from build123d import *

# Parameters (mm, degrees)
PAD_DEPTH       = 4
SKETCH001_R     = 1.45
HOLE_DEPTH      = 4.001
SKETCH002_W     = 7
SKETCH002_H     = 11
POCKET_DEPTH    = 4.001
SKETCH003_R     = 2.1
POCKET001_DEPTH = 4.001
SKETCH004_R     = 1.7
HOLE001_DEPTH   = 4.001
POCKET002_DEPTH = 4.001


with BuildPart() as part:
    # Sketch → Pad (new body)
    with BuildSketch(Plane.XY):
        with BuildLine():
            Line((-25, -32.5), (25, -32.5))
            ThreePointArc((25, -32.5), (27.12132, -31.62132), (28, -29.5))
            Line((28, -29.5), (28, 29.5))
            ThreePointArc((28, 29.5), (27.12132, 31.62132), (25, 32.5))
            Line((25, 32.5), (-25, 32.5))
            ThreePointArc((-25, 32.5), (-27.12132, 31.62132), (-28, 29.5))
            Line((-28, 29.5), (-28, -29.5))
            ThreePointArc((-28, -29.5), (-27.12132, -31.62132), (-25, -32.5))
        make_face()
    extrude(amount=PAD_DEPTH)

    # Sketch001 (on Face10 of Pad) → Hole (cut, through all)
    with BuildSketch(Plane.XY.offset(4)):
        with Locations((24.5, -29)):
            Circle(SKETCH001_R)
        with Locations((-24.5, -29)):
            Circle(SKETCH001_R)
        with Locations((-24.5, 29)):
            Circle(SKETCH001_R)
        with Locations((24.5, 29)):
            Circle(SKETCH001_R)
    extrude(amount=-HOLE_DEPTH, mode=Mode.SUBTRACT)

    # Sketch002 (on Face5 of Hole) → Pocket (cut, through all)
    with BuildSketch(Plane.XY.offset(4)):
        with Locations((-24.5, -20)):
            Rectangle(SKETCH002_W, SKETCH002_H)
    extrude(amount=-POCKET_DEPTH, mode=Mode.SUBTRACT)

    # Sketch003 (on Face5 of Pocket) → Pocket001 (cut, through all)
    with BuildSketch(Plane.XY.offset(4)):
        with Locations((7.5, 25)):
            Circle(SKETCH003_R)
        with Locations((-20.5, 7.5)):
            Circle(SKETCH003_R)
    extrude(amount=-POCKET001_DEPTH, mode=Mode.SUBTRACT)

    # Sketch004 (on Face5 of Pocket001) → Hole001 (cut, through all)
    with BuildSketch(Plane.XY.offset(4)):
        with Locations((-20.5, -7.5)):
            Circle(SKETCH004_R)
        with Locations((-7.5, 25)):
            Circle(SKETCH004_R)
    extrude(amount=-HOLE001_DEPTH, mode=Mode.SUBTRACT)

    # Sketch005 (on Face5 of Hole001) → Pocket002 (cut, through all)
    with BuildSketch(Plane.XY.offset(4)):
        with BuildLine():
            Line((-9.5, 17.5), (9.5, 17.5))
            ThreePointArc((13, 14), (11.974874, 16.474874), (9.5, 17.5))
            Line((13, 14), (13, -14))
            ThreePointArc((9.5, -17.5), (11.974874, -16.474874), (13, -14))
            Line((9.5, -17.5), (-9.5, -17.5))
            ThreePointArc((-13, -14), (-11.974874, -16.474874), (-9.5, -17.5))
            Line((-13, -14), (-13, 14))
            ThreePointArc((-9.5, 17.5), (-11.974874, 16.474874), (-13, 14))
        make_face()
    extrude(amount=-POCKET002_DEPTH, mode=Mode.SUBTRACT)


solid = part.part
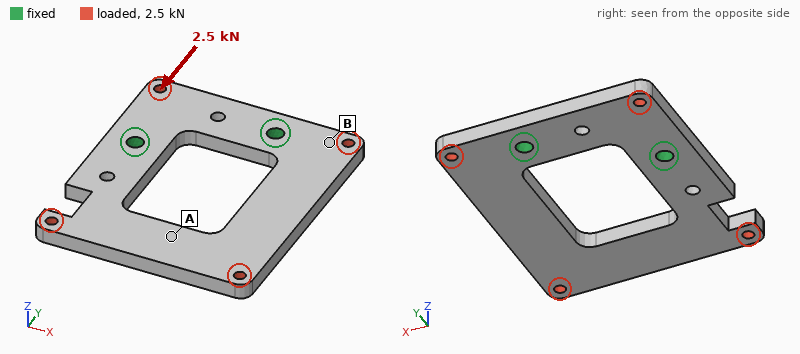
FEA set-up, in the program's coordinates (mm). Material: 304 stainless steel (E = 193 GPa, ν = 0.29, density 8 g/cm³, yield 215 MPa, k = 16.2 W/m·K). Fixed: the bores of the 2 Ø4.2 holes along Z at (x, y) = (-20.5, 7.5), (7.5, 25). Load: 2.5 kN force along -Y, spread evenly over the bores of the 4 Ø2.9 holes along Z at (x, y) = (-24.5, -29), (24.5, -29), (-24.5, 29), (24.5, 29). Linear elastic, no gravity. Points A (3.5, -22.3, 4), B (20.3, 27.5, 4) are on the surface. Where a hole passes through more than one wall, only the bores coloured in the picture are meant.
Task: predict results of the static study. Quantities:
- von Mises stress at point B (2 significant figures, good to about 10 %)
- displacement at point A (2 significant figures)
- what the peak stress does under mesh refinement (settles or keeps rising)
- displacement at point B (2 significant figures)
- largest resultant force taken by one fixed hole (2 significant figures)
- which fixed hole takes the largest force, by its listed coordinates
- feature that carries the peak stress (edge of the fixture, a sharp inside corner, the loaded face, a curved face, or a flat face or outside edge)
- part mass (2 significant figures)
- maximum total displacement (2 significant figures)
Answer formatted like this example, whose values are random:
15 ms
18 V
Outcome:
19 MPa
13 µm
keeps rising
8.1 µm
1.4 kN
(7.5, 25)
edge of the fixture
83 g
19 µm
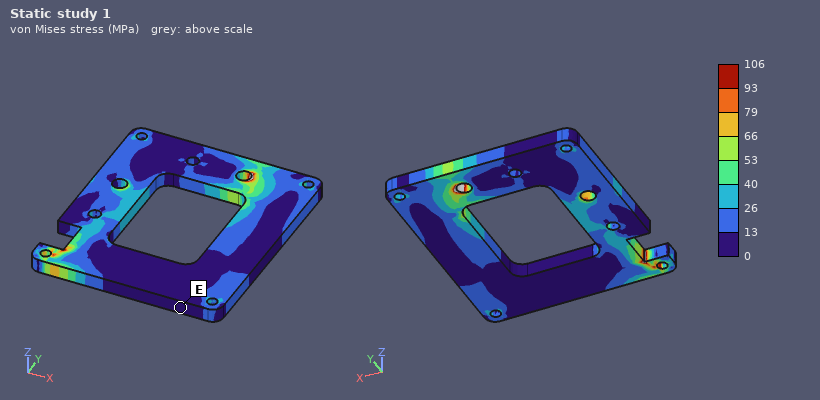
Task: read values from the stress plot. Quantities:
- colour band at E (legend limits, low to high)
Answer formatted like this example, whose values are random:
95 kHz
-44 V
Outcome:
0 to 13 MPa
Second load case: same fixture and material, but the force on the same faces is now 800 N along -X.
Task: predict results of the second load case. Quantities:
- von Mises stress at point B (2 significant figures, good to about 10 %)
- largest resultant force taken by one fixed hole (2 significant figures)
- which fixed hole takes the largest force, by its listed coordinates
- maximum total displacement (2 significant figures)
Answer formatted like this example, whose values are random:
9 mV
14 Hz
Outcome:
9.0 MPa
530 N
(-20.5, 7.5)
14 µm
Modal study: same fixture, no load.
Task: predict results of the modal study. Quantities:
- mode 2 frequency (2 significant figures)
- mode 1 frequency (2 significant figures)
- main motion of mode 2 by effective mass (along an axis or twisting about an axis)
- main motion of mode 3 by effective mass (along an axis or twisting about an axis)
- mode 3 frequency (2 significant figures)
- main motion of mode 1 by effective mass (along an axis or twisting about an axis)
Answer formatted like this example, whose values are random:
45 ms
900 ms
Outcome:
2500 Hz
980 Hz
twisting about Y
along X
4800 Hz
along Z
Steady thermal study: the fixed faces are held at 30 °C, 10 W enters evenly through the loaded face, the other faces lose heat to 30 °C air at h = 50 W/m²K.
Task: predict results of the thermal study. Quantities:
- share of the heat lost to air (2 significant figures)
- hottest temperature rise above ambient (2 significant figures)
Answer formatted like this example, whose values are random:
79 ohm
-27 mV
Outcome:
64 %
74 K
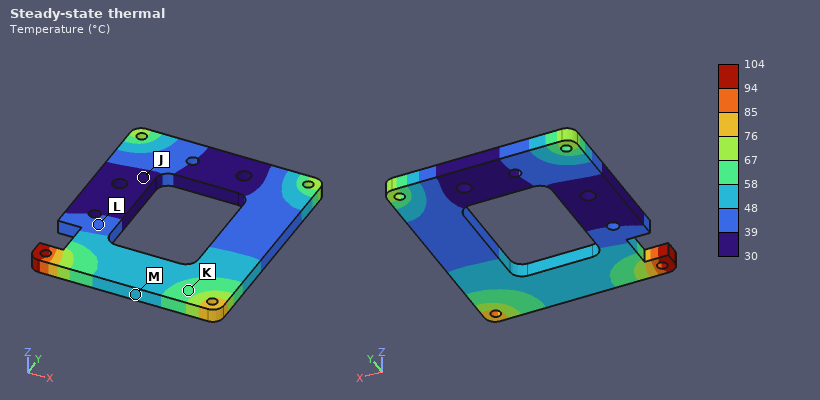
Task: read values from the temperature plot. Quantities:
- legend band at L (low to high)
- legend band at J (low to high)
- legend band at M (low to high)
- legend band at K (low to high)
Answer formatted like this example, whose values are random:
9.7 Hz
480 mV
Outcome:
39 to 48 °C
30 to 39 °C
48 to 58 °C
58 to 67 °C
